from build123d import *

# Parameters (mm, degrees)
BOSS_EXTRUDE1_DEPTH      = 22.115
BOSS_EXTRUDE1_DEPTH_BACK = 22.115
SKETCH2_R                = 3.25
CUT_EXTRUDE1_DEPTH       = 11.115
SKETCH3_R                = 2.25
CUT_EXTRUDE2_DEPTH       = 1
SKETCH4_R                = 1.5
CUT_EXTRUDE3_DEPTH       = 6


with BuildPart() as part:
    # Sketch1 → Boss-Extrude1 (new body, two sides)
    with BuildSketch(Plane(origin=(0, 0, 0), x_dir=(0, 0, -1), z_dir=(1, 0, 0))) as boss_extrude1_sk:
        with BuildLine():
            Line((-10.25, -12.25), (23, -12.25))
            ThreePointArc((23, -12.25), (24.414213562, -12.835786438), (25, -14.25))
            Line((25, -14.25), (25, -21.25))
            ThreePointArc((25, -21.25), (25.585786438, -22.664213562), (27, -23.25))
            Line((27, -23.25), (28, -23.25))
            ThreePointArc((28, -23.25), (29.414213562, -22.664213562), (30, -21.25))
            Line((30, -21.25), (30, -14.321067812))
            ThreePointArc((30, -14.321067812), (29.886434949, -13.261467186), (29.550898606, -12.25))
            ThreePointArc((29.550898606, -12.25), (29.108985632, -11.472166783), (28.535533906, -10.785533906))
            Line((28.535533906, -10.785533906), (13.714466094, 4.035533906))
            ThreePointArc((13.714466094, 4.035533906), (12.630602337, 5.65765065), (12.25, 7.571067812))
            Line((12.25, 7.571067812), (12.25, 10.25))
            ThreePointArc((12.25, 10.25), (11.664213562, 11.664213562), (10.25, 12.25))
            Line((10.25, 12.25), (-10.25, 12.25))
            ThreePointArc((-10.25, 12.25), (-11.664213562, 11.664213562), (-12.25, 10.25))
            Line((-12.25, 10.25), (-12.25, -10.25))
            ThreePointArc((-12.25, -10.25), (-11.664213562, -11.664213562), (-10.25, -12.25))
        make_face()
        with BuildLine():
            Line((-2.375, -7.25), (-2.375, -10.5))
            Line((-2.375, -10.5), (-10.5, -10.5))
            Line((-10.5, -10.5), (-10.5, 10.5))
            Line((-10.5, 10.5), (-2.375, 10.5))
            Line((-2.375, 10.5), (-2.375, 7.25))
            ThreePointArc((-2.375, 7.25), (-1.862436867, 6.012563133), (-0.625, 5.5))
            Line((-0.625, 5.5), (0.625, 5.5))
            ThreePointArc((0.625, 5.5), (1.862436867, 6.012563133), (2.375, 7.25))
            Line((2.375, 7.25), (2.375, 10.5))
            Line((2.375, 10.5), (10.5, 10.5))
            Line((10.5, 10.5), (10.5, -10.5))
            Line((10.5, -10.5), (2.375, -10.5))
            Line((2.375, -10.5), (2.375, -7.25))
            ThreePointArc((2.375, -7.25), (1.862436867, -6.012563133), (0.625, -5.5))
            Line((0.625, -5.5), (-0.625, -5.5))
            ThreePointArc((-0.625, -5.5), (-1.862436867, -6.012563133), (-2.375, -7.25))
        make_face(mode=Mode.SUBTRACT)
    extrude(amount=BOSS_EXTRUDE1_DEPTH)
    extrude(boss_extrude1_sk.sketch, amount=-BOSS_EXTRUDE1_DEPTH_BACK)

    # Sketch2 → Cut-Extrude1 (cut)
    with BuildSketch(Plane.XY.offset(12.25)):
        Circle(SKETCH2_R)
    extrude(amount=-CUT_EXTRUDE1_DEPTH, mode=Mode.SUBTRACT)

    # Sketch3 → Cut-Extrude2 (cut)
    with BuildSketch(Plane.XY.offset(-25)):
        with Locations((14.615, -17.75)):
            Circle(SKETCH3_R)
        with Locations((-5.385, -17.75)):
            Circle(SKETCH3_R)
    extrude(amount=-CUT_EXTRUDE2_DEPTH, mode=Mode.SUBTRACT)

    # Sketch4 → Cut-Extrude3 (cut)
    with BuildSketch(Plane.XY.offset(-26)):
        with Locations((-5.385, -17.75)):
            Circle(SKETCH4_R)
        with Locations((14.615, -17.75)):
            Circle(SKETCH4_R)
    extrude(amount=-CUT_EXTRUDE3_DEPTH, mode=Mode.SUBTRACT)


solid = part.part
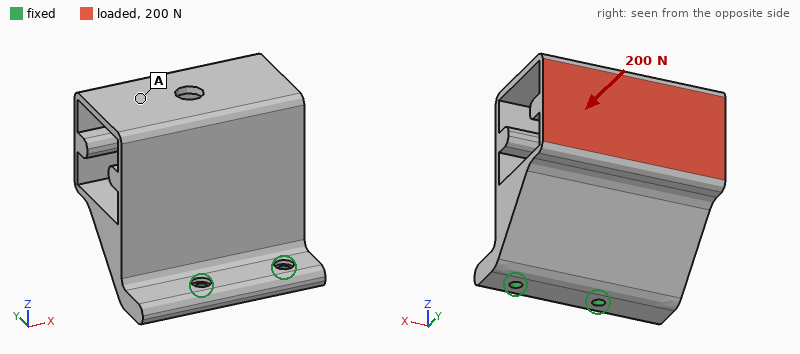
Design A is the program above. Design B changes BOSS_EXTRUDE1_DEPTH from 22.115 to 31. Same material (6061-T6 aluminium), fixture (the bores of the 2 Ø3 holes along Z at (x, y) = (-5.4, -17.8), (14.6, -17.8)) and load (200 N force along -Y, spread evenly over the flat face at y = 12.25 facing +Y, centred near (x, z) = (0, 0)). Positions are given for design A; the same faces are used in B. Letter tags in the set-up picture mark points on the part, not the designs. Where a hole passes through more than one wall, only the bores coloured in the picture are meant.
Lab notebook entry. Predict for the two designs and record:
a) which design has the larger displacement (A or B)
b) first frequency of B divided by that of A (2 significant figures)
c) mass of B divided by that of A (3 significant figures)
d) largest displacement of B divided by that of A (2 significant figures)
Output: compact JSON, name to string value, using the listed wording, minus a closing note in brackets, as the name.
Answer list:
{"which design has the larger displacement": "A", "first frequency of B divided by that of A": "0.97", "mass of B divided by that of A": "1.20", "largest displacement of B divided by that of A": "0.87"}
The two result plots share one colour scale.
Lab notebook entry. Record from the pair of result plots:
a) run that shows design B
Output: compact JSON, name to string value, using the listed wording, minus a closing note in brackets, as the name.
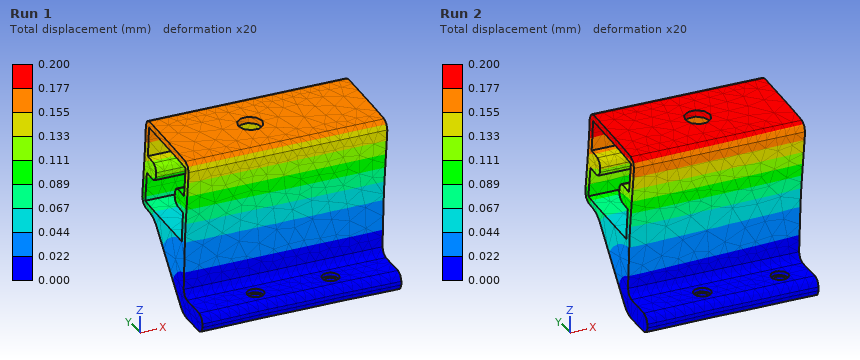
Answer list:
{"run that shows design B": "Run 1"}
